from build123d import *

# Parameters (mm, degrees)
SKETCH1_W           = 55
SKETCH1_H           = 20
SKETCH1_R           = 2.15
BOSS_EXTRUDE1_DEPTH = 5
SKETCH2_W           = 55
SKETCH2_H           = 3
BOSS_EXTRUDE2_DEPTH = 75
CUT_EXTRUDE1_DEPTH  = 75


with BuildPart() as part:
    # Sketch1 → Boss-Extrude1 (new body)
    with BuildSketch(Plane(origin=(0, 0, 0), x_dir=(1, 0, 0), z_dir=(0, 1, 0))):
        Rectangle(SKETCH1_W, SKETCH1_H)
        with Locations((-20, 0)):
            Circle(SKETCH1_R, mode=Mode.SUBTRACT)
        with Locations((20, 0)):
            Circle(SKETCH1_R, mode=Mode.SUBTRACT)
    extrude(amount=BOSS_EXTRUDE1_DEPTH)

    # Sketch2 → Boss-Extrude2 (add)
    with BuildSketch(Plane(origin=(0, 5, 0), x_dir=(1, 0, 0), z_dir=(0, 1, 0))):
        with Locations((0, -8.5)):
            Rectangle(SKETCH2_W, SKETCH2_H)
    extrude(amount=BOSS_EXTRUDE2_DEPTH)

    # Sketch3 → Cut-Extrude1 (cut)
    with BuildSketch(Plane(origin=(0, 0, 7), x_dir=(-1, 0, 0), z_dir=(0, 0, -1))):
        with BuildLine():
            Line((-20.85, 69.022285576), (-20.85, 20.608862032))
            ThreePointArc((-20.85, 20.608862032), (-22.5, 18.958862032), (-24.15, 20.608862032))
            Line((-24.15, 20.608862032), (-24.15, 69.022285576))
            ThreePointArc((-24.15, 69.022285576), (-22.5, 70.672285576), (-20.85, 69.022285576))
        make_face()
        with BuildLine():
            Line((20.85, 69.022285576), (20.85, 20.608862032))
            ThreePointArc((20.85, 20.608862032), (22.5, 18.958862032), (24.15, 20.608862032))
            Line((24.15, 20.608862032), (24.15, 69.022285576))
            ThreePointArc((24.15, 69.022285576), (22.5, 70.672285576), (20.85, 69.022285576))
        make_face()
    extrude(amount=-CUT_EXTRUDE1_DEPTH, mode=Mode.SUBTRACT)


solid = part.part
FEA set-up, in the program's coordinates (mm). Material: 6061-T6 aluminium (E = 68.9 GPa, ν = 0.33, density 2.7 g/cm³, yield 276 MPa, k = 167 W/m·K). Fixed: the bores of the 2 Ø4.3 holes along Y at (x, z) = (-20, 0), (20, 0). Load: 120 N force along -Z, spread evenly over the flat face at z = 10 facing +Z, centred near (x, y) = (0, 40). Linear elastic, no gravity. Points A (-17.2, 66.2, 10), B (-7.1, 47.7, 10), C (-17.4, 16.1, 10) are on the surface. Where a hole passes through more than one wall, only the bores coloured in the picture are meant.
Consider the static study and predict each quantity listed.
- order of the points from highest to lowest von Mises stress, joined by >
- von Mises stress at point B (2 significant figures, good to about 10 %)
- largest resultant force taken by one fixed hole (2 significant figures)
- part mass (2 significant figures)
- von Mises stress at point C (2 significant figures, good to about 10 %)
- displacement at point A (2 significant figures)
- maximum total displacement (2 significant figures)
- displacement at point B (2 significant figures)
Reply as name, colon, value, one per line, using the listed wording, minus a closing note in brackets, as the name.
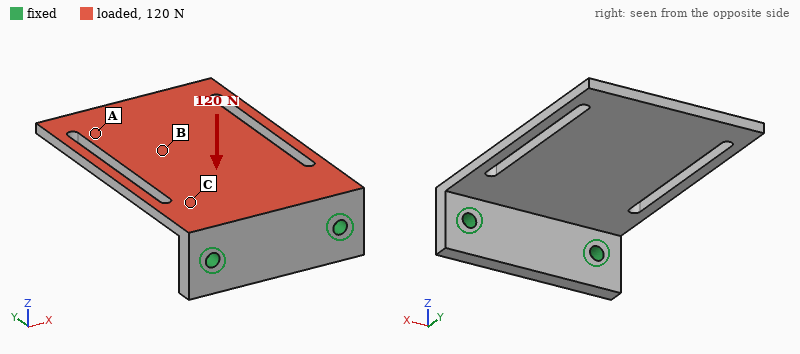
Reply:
order of the points from highest to lowest von Mises stress, joined by >: C > B > A
von Mises stress at point B: 11 MPa
largest resultant force taken by one fixed hole: 61 N
part mass: 45 g
von Mises stress at point C: 36 MPa
displacement at point A: 0.63 mm
maximum total displacement: 0.83 mm
displacement at point B: 0.38 mm
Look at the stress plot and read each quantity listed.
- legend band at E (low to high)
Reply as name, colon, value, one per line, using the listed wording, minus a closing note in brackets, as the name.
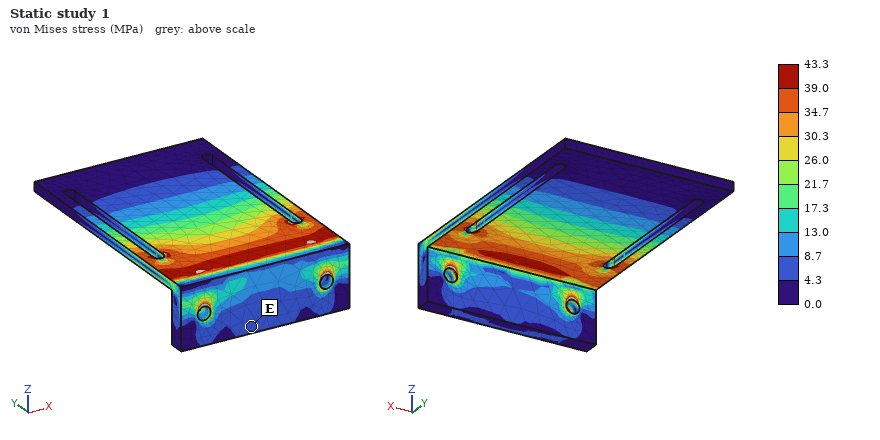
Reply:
legend band at E: 4.3 to 8.7 MPa
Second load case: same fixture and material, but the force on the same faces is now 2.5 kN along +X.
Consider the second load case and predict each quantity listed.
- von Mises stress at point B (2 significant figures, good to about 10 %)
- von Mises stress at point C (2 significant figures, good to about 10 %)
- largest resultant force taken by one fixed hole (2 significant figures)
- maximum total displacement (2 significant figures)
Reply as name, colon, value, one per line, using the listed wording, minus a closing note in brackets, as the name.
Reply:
von Mises stress at point B: 36 MPa
von Mises stress at point C: 30 MPa
largest resultant force taken by one fixed hole: 2.6 kN
maximum total displacement: 0.28 mm
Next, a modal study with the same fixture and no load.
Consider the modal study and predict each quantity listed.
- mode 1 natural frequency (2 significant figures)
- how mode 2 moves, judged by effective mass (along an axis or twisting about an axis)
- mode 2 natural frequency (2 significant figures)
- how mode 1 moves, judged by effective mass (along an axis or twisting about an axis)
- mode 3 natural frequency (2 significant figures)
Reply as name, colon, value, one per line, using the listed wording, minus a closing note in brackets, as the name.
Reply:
mode 1 natural frequency: 410 Hz
how mode 2 moves, judged by effective mass: twisting about Y
mode 2 natural frequency: 1300 Hz
how mode 1 moves, judged by effective mass: along Z
mode 3 natural frequency: 2500 Hz
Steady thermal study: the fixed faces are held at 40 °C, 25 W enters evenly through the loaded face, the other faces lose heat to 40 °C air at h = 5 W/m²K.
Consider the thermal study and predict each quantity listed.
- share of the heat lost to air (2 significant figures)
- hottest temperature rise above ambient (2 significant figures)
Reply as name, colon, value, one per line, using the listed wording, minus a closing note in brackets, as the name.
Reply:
share of the heat lost to air: 3.2 %
hottest temperature rise above ambient: 41 K
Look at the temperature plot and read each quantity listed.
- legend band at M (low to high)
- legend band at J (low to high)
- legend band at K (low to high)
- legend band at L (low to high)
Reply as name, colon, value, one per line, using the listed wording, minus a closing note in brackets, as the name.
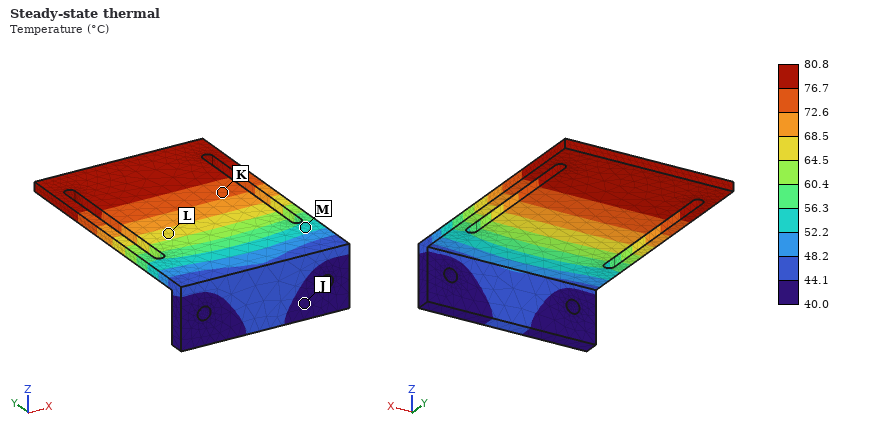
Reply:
legend band at M: 52.2 to 56.3 °C
legend band at J: 40.0 to 44.1 °C
legend band at K: 72.6 to 76.7 °C
legend band at L: 64.5 to 68.5 °C
